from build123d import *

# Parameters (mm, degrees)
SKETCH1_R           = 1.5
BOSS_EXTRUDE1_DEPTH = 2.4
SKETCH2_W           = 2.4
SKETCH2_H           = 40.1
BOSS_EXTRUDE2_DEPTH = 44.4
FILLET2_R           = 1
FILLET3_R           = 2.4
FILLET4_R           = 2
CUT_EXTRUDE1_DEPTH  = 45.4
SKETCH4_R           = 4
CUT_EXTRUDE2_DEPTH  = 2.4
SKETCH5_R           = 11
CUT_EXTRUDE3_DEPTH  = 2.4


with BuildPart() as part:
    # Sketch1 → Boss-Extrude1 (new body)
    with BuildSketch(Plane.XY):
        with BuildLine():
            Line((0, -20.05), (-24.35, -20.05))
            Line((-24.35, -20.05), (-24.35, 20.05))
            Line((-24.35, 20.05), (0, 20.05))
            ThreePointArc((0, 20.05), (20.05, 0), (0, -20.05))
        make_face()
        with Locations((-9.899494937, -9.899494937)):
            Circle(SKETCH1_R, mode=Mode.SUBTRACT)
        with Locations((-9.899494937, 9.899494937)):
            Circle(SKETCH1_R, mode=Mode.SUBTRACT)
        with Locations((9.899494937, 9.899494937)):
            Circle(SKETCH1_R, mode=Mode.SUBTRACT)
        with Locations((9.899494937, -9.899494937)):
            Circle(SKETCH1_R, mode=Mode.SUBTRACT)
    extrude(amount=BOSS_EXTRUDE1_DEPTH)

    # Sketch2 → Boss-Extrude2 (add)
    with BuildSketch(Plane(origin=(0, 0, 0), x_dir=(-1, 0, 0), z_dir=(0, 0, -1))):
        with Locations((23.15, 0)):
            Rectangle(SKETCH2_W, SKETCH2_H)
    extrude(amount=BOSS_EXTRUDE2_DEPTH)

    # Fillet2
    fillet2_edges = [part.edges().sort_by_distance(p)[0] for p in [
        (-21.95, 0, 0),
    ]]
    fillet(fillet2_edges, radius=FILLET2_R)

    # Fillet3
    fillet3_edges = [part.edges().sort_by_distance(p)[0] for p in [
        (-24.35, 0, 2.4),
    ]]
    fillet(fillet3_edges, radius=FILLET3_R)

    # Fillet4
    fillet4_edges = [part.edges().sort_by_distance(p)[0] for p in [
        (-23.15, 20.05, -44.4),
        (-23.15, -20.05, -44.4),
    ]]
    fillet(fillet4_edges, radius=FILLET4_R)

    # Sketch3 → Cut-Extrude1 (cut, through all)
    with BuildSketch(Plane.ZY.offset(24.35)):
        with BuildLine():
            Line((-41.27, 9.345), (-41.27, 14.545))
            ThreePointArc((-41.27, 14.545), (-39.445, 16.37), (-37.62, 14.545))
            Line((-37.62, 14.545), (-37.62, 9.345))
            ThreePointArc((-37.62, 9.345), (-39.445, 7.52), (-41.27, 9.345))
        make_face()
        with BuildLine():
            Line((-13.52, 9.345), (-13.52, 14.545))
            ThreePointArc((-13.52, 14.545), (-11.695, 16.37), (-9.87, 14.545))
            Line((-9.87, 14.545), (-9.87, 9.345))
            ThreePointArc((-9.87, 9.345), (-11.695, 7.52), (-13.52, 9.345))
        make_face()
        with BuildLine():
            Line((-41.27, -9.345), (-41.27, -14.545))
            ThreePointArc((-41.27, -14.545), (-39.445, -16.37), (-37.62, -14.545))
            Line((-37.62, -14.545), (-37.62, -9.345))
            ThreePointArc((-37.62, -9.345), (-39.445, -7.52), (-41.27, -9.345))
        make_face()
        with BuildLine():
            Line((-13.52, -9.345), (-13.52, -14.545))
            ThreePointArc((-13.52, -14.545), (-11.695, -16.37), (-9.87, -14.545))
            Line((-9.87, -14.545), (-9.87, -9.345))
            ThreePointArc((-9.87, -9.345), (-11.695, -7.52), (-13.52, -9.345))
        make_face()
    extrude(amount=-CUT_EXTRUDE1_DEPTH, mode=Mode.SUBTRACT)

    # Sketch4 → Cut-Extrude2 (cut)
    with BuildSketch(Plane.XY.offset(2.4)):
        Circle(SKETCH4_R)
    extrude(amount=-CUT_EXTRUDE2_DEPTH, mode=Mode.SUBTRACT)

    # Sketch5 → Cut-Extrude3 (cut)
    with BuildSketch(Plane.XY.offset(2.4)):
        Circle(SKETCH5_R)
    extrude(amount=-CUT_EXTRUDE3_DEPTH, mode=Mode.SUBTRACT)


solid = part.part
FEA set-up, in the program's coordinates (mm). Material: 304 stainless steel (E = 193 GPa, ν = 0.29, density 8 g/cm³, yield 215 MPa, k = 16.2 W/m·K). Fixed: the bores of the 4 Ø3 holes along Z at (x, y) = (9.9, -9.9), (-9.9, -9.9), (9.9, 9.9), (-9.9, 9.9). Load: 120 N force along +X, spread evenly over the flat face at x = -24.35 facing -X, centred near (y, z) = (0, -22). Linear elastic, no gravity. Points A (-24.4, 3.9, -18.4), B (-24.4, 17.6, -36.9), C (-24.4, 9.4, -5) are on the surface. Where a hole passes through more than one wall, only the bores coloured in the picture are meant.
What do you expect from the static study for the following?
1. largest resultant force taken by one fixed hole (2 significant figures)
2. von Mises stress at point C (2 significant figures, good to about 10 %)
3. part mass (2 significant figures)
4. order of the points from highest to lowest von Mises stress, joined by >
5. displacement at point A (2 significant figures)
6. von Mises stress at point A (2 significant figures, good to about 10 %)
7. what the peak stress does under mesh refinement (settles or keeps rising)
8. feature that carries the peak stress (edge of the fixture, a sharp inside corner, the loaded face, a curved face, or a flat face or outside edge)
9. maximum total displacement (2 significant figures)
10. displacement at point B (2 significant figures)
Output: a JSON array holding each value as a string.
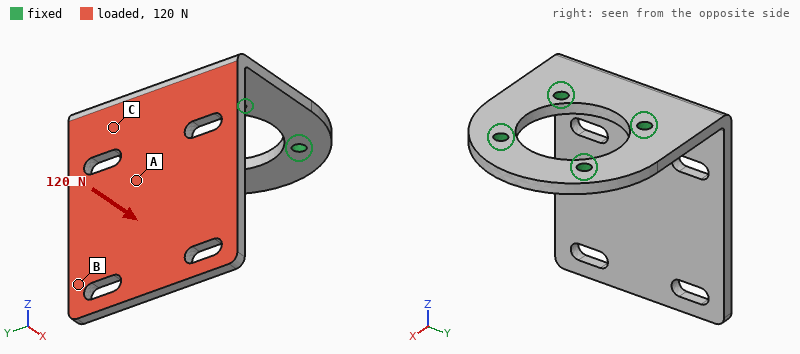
["64 N", "45 MPa", "55 g", "C > A > B", "0.13 mm", "25 MPa", "keeps rising", "edge of the fixture", "0.36 mm", "0.29 mm"]
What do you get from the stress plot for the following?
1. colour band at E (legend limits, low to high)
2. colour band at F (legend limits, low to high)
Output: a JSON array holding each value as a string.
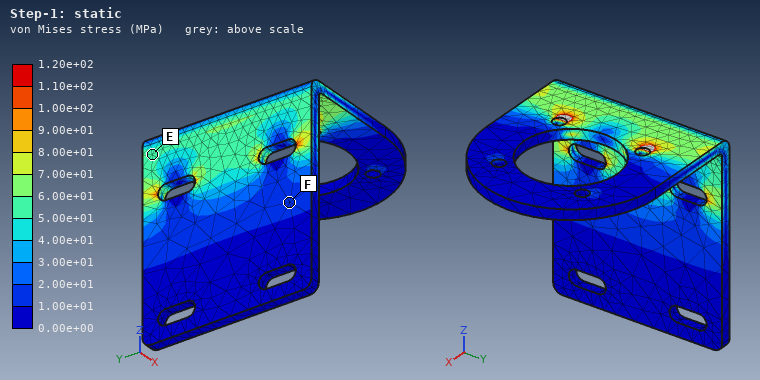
["5.00e+01 to 6.00e+01 MPa", "1.00e+01 to 2.00e+01 MPa"]
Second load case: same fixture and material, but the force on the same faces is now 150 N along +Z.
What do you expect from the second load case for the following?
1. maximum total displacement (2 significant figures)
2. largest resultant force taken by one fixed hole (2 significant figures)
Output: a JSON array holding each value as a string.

["0.11 mm", "83 N"]
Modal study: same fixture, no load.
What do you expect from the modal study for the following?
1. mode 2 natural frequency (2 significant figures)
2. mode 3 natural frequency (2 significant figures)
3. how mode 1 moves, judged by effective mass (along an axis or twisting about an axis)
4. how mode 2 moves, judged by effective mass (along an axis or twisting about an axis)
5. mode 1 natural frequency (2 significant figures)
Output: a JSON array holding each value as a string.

["1600 Hz", "2500 Hz", "along X", "along Y", "630 Hz"]
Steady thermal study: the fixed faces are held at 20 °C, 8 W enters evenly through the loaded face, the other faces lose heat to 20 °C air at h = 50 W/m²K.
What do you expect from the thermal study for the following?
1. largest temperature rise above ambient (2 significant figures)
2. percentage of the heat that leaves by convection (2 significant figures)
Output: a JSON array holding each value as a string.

["57 K", "75 %"]
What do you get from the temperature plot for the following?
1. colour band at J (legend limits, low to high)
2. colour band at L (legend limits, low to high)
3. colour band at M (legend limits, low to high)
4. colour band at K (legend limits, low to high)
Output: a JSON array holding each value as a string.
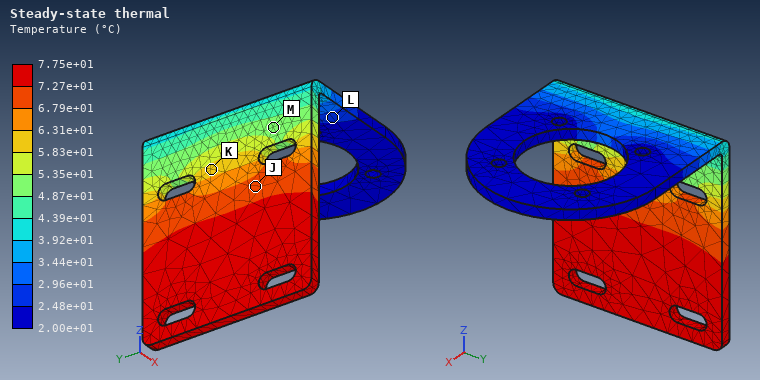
["6.79e+01 to 7.27e+01 °C", "2.48e+01 to 2.96e+01 °C", "4.87e+01 to 5.35e+01 °C", "5.83e+01 to 6.31e+01 °C"]
